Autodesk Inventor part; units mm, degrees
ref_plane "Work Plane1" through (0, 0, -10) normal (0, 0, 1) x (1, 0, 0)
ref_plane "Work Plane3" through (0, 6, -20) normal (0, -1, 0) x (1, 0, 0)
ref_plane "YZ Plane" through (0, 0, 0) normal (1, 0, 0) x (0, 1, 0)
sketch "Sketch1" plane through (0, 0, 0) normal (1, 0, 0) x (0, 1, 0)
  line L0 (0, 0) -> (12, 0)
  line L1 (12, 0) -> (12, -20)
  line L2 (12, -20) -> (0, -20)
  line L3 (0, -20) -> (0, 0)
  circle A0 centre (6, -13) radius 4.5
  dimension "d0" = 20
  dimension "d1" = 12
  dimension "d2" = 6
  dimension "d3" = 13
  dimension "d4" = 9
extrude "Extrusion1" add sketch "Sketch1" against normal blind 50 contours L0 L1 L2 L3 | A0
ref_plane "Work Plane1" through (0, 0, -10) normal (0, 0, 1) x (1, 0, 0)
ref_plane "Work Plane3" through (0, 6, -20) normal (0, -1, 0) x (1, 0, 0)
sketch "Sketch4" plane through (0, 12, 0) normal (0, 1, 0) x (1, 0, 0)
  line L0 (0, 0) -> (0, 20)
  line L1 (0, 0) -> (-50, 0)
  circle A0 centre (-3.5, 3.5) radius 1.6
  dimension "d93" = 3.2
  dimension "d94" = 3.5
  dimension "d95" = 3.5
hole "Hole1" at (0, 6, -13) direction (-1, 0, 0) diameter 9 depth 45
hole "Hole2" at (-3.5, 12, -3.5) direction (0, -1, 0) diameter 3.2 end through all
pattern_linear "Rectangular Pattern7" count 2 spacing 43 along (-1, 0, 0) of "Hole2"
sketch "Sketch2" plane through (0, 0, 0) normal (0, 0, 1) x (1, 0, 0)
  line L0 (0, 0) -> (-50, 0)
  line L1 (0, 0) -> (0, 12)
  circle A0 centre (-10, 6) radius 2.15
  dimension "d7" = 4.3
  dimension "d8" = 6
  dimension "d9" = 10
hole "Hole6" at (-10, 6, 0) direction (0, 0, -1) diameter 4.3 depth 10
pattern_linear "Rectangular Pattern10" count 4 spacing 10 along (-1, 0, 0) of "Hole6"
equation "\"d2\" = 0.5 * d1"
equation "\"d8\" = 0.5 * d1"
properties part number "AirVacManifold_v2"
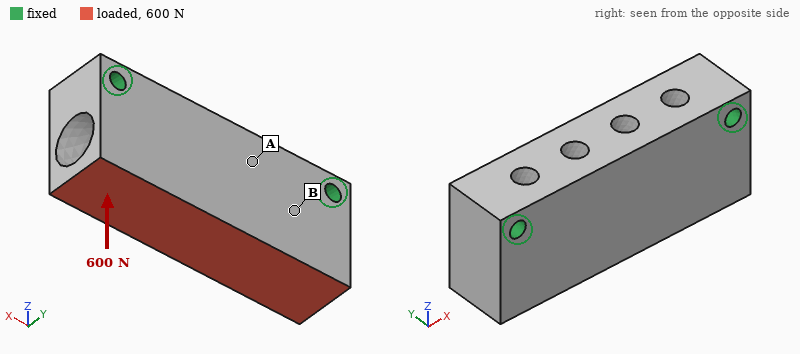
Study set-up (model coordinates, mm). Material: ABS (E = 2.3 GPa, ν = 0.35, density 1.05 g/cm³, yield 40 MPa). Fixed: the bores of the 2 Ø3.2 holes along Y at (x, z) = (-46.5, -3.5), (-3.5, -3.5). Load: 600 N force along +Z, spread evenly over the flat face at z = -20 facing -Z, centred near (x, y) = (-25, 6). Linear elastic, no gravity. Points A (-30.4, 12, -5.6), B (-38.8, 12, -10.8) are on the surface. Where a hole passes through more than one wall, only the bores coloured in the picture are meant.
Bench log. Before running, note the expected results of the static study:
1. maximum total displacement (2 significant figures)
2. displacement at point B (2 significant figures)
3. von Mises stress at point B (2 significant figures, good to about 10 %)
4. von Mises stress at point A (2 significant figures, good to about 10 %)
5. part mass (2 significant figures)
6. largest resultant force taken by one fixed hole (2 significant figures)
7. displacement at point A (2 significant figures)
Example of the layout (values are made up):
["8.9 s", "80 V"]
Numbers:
["76 µm", "33 µm", "5.2 MPa", "1.7 MPa", "8.9 g", "330 N", "47 µm"]
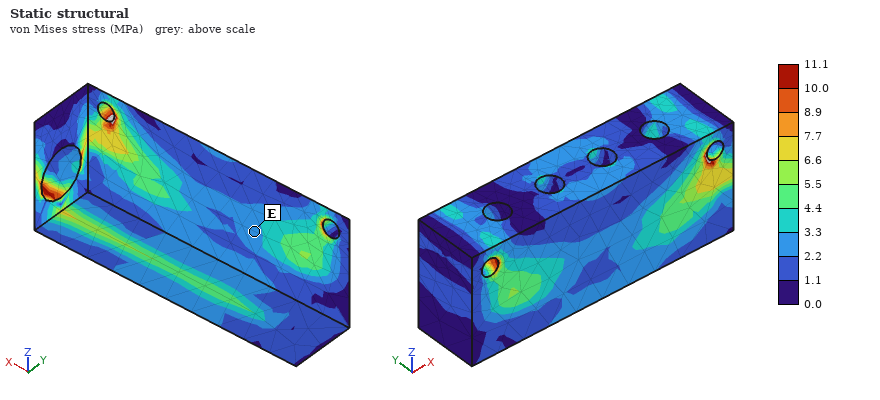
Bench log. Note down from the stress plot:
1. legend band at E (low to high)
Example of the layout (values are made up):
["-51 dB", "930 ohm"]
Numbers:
["2.2 to 3.3 MPa"]
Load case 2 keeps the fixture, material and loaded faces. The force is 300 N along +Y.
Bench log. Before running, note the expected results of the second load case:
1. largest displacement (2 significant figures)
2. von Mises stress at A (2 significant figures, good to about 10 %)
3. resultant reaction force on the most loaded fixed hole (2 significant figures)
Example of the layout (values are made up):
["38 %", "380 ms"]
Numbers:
["0.22 mm", "2.6 MPa", "150 N"]
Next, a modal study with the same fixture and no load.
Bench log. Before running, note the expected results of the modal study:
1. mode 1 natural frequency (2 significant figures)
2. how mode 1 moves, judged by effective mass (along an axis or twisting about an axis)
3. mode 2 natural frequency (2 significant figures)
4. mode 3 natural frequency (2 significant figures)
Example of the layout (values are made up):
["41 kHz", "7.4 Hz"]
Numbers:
["3900 Hz", "along Y", "6400 Hz", "6500 Hz"]
